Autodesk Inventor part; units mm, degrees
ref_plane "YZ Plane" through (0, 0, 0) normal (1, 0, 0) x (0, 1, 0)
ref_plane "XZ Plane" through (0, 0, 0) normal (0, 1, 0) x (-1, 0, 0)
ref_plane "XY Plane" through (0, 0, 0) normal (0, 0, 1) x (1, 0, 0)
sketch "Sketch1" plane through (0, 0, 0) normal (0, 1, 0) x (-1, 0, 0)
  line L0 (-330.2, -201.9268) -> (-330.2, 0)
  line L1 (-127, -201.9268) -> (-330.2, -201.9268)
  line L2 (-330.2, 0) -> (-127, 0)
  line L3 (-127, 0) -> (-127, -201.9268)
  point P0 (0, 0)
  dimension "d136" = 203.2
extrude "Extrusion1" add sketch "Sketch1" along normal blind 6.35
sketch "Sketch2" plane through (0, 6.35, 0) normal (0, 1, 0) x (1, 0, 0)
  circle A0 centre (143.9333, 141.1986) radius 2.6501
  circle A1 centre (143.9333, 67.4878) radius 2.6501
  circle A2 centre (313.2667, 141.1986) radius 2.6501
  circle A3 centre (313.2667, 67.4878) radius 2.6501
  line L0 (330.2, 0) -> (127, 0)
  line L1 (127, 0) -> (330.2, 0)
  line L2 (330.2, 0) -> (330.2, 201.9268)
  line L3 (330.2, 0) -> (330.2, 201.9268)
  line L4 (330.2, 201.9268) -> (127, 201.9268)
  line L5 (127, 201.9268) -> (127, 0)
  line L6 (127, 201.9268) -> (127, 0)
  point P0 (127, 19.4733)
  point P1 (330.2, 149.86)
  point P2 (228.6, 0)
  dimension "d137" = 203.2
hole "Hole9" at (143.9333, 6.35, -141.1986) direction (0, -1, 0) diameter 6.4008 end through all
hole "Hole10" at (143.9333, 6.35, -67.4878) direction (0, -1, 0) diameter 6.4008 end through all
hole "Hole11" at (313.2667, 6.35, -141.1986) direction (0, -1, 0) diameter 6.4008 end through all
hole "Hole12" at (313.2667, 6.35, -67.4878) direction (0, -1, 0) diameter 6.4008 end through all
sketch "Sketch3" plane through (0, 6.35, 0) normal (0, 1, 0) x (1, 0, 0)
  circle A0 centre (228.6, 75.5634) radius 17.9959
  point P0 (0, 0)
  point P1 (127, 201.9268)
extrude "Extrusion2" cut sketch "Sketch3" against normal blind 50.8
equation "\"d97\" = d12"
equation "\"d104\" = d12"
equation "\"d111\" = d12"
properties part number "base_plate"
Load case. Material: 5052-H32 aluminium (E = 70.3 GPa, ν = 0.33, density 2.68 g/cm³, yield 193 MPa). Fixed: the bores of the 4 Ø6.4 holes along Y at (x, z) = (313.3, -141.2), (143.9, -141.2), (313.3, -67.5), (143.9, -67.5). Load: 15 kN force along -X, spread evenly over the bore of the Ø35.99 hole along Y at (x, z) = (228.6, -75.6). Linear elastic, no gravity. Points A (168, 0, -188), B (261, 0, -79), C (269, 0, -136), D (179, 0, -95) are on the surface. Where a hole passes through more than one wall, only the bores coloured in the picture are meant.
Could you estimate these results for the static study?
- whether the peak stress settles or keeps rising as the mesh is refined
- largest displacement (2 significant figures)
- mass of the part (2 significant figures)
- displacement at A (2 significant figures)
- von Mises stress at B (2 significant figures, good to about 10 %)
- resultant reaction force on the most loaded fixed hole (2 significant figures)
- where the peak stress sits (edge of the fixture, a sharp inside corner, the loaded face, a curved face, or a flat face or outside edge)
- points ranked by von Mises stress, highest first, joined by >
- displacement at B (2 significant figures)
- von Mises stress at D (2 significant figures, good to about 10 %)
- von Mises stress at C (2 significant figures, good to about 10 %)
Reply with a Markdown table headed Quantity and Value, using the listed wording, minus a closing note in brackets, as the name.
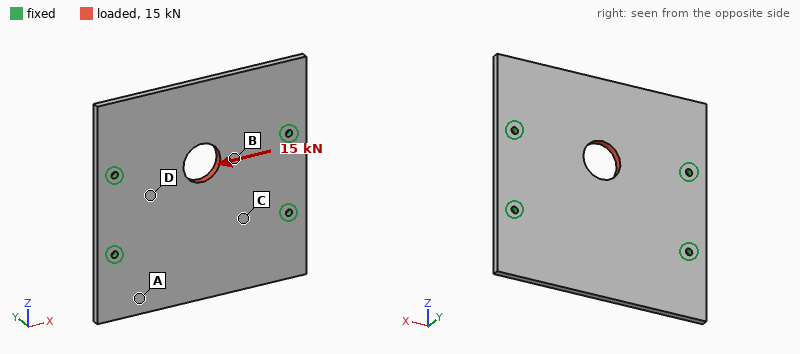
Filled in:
| Quantity | Value |
|---|---|
| whether the peak stress settles or keeps rising as the mesh is refined | keeps rising |
| largest displacement | 24 µm |
| mass of the part | 680 g |
| displacement at A | 4.0 µm |
| von Mises stress at B | 20 MPa |
| resultant reaction force on the most loaded fixed hole | 5.1 kN |
| where the peak stress sits | edge of the fixture |
| points ranked by von Mises stress, highest first, joined by > | B > D > C > A |
| displacement at B | 16 µm |
| von Mises stress at D | 11 MPa |
| von Mises stress at C | 5.6 MPa |
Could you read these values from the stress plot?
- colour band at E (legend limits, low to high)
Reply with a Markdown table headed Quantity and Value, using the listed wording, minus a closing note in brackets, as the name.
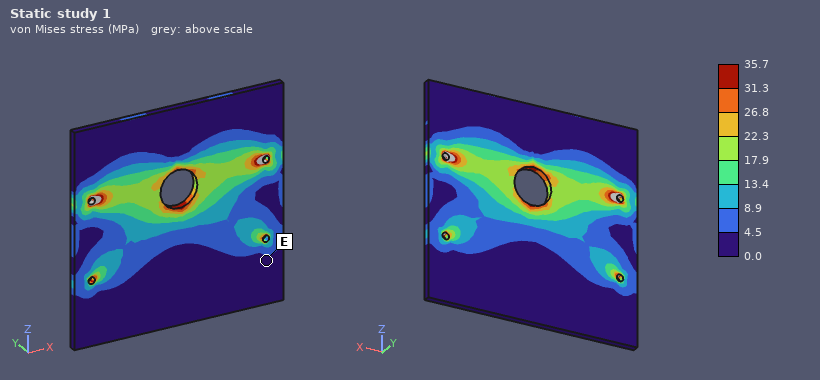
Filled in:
| Quantity | Value |
|---|---|
| colour band at E | 0.0 to 4.5 MPa |
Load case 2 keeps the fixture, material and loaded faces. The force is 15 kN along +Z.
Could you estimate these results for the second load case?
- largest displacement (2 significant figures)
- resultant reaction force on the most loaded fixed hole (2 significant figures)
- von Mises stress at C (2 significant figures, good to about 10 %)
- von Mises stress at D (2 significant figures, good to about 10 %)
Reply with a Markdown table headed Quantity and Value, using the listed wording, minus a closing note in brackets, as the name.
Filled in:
| Quantity | Value |
|---|---|
| largest displacement | 36 µm |
| resultant reaction force on the most loaded fixed hole | 3.9 kN |
| von Mises stress at C | 11 MPa |
| von Mises stress at D | 15 MPa |
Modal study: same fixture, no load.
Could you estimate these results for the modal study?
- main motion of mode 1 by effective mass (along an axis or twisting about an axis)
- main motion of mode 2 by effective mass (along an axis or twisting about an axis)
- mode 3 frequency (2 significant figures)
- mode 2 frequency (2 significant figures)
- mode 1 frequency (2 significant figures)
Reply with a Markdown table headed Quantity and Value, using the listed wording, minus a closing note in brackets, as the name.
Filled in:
| Quantity | Value |
|---|---|
| main motion of mode 1 by effective mass | along Y |
| main motion of mode 2 by effective mass | along Y |
| mode 3 frequency | 1300 Hz |
| mode 2 frequency | 810 Hz |
| mode 1 frequency | 720 Hz |
